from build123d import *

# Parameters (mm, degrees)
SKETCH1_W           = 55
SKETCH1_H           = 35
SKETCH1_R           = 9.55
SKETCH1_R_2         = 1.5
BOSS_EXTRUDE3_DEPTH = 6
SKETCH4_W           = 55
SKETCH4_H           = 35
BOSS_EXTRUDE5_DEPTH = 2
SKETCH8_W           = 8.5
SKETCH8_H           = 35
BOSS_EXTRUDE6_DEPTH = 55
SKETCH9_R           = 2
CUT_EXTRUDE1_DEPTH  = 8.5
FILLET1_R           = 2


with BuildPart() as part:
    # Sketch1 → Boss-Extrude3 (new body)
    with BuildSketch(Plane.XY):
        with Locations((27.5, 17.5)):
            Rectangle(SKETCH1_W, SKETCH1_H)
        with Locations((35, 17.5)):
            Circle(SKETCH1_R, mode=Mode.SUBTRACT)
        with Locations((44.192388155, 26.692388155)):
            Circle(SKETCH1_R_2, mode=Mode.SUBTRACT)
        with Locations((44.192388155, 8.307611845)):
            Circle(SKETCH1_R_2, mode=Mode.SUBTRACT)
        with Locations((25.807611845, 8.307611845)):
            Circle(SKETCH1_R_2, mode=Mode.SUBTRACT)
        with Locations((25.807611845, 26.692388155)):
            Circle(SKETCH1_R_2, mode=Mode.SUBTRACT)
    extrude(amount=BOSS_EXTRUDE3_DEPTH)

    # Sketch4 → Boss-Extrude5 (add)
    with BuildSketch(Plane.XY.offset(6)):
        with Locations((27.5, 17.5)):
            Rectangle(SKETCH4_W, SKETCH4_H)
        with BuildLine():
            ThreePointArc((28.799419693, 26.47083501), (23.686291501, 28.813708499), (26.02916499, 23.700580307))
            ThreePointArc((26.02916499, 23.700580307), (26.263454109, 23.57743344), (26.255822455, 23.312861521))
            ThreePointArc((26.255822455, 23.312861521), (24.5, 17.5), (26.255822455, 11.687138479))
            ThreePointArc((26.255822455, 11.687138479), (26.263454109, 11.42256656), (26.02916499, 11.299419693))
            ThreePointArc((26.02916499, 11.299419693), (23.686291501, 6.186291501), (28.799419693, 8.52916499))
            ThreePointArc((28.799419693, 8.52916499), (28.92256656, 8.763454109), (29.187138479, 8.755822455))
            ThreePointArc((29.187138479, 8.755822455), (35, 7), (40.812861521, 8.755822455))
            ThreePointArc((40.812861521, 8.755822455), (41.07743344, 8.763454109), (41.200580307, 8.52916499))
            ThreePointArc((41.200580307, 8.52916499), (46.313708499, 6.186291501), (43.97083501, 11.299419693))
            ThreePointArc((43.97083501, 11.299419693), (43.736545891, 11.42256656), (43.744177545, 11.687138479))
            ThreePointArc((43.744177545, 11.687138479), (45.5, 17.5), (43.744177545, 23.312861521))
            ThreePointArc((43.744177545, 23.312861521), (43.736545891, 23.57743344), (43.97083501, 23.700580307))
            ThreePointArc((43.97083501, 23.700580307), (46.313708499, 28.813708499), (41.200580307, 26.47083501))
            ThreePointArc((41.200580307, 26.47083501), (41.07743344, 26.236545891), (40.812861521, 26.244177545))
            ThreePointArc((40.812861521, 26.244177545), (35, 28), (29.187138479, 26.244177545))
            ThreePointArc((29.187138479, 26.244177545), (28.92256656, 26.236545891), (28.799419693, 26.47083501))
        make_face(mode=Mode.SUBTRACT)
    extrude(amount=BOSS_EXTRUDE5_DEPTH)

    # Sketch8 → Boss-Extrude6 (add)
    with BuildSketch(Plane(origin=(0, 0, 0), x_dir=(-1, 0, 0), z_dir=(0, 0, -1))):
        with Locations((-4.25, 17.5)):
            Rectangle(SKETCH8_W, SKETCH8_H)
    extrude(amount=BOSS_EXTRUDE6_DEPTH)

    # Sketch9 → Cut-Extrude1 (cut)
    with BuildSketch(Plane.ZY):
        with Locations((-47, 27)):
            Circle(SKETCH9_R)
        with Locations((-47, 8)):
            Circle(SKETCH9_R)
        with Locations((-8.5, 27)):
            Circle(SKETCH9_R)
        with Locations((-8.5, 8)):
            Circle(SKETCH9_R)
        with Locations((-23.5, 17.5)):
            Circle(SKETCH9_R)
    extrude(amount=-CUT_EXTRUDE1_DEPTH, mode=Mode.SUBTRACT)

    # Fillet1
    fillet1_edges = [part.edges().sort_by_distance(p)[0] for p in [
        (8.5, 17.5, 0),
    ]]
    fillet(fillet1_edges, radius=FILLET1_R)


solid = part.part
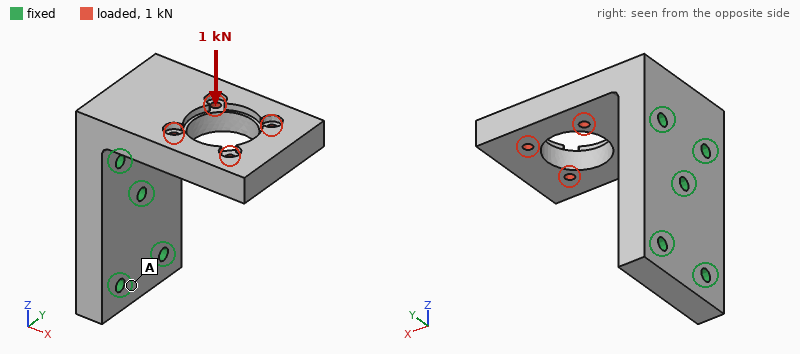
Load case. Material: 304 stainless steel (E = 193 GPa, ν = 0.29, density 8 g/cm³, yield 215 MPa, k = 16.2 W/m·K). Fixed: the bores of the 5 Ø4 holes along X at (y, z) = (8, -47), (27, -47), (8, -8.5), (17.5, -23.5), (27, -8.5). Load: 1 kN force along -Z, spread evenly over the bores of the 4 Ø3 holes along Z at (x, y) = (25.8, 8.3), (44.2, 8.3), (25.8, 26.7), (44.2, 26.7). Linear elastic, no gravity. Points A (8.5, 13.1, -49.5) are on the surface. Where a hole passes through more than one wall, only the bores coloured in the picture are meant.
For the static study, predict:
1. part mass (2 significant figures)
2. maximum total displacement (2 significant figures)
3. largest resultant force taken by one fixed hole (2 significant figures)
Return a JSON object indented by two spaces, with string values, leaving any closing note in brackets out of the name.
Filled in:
{
  "part mass": "230 g",
  "maximum total displacement": "0.13 mm",
  "largest resultant force taken by one fixed hole": "520 N"
}
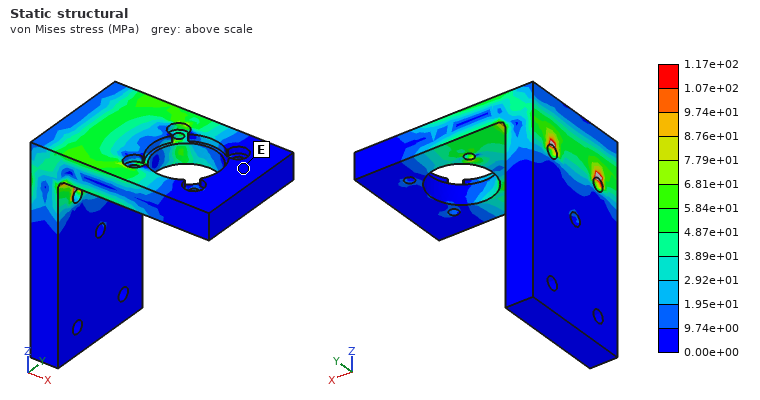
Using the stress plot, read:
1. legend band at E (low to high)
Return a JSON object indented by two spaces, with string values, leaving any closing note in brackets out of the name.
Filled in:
{
  "legend band at E": "0.00e+00 to 9.74e+00 MPa"
}
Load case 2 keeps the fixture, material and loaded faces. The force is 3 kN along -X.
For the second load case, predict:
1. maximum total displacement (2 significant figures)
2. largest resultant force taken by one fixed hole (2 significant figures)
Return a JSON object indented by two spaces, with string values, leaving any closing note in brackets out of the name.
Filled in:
{
  "maximum total displacement": "26 µm",
  "largest resultant force taken by one fixed hole": "1.7 kN"
}
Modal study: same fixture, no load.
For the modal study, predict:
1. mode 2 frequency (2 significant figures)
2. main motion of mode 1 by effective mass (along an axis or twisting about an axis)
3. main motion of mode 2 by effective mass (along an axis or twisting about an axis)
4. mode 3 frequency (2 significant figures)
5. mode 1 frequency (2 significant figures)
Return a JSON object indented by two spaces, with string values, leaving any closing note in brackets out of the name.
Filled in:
{
  "mode 2 frequency": "4300 Hz",
  "main motion of mode 1 by effective mass": "along Z",
  "main motion of mode 2 by effective mass": "along Y",
  "mode 3 frequency": "5800 Hz",
  "mode 1 frequency": "2000 Hz"
}
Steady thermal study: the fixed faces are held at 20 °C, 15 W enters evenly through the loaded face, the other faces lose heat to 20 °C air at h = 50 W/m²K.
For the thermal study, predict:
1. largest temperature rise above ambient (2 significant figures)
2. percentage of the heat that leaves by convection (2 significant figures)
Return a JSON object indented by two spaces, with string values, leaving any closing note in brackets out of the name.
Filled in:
{
  "largest temperature rise above ambient": "68 K",
  "percentage of the heat that leaves by convection": "66 %"
}
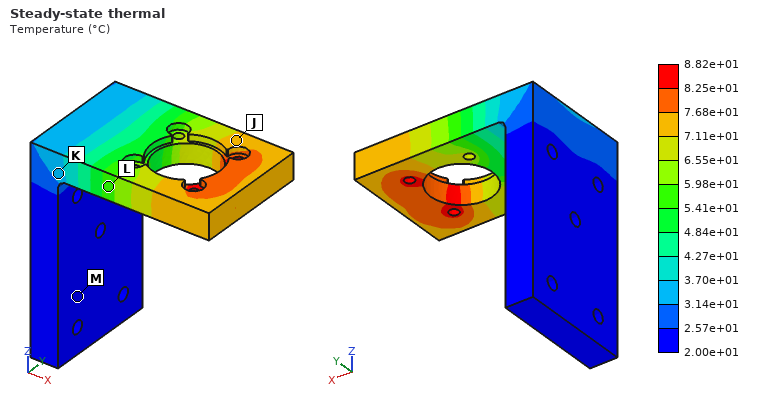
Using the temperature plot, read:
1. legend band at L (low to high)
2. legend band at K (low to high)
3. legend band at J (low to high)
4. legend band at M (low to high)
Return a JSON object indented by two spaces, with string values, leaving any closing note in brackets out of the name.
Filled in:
{
  "legend band at L": "5.41e+01 to 5.98e+01 °C",
  "legend band at K": "3.14e+01 to 3.70e+01 °C",
  "legend band at J": "7.11e+01 to 7.68e+01 °C",
  "legend band at M": "2.00e+01 to 2.57e+01 °C"
}
